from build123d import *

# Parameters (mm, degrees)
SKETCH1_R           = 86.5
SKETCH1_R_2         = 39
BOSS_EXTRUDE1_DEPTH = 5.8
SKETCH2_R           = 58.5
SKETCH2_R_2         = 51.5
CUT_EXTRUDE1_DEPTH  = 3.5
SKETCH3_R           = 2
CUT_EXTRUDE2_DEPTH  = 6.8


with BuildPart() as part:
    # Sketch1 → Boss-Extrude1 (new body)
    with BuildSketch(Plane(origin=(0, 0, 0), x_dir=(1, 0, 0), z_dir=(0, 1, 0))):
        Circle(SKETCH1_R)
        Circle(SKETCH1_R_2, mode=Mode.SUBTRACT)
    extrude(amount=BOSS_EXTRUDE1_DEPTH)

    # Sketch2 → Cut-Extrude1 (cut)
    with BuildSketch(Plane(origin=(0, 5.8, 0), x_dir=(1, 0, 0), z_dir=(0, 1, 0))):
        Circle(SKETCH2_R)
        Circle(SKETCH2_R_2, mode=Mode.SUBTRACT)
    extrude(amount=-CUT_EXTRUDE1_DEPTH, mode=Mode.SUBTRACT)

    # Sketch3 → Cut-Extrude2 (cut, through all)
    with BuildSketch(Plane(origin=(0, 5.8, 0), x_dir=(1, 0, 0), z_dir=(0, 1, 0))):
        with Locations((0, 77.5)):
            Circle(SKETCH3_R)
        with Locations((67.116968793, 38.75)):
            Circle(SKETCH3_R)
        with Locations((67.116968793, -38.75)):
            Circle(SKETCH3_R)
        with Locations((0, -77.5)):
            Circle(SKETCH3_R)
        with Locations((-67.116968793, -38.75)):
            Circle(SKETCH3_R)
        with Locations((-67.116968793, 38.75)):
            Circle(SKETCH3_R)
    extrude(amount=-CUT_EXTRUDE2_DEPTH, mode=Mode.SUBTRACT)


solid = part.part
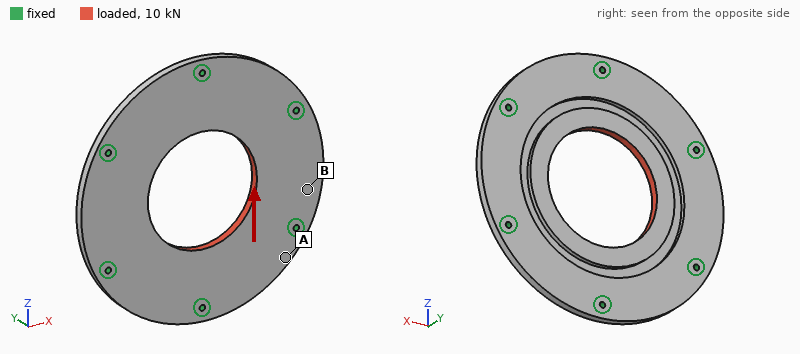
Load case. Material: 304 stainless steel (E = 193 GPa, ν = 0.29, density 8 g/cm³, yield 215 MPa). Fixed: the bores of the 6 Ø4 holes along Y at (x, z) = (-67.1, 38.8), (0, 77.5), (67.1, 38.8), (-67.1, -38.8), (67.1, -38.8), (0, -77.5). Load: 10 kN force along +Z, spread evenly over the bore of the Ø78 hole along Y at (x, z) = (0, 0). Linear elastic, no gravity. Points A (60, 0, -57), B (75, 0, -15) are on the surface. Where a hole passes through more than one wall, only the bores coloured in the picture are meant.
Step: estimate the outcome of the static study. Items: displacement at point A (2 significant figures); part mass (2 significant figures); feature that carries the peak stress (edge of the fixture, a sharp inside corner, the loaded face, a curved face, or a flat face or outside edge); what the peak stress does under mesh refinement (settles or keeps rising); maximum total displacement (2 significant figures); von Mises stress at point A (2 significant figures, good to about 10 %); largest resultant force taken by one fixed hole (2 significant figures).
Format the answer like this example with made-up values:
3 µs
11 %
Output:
2.1 µm
800 g
edge of the fixture
keeps rising
7.8 µm
7.2 MPa
2.0 kN
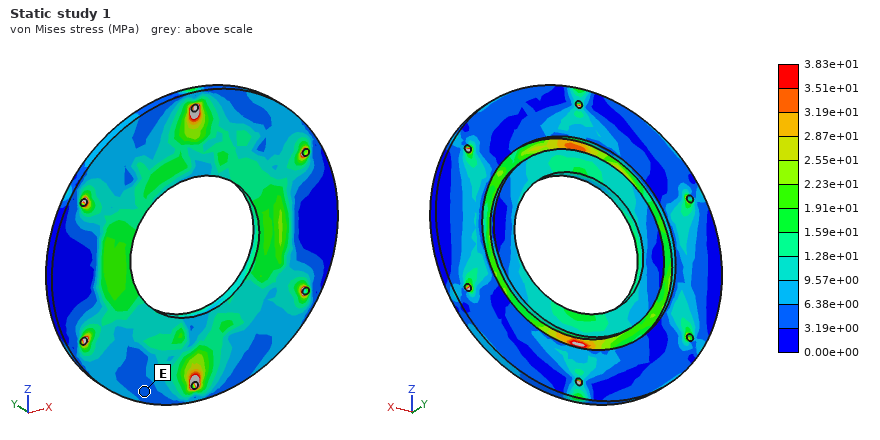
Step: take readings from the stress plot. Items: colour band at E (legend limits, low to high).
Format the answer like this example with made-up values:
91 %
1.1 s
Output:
3.19e+00 to 6.38e+00 MPa
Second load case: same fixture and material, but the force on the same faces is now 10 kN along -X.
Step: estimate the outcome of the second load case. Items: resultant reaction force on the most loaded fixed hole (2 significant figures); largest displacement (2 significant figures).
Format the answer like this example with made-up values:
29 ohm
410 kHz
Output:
1.9 kN
7.9 µm
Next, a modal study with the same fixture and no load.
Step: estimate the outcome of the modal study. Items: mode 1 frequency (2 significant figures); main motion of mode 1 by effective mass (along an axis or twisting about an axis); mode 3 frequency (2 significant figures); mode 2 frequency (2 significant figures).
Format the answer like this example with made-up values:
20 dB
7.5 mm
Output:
2600 Hz
along Y
3400 Hz
3400 Hz
